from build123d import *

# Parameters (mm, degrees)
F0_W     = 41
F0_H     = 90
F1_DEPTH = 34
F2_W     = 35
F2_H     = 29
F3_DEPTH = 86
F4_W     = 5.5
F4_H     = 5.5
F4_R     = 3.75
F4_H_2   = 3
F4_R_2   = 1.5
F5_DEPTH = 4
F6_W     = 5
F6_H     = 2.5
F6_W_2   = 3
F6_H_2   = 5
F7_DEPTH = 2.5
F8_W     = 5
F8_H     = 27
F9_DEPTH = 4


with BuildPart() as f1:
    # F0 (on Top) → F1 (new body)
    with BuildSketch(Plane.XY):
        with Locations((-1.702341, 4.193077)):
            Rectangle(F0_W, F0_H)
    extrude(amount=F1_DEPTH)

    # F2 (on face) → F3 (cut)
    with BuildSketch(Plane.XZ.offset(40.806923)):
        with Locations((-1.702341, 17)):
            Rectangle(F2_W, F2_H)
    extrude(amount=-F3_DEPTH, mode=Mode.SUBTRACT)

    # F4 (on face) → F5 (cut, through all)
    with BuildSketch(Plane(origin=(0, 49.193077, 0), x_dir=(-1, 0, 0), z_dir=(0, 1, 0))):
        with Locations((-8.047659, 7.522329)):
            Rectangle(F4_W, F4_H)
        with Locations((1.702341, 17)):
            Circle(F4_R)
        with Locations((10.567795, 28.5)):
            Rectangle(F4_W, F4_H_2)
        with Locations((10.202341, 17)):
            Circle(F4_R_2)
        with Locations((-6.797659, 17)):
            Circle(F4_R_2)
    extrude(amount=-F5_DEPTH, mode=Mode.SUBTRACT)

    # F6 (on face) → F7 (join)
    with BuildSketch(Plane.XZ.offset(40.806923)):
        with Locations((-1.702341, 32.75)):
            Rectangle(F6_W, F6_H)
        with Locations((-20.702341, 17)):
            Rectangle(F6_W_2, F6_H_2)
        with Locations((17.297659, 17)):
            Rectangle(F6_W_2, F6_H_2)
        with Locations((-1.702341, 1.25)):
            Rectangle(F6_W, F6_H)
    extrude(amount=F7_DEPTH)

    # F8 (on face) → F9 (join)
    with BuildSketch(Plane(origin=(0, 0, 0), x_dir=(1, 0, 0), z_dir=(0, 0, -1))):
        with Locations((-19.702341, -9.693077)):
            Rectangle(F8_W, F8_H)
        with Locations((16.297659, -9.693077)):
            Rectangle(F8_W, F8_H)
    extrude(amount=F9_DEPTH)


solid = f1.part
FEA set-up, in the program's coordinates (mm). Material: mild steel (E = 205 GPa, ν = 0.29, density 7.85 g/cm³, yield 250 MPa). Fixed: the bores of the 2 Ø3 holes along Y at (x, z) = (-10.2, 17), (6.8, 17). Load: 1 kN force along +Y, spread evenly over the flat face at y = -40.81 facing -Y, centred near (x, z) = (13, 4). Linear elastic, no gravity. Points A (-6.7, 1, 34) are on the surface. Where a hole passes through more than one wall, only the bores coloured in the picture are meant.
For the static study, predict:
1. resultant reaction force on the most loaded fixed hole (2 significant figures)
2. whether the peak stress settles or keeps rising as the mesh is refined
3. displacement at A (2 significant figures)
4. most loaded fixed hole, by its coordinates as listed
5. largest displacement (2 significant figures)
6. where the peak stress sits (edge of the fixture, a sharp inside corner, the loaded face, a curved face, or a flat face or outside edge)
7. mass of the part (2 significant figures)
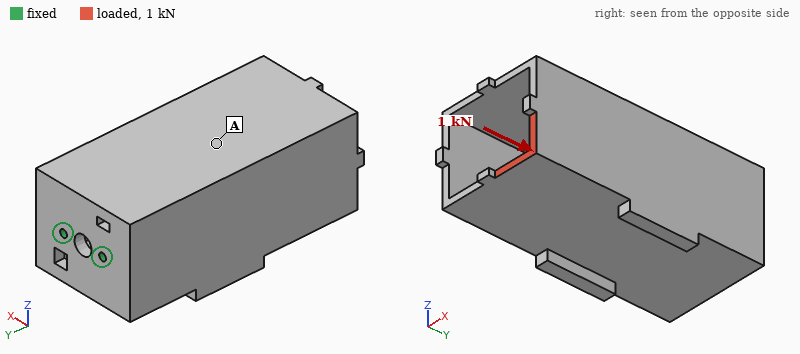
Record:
1.1 kN
keeps rising
0.061 mm
(6.8, 17)
0.12 mm
edge of the fixture
310 g
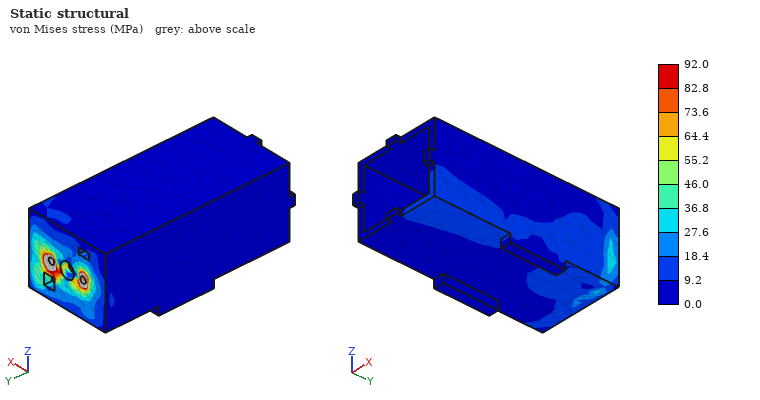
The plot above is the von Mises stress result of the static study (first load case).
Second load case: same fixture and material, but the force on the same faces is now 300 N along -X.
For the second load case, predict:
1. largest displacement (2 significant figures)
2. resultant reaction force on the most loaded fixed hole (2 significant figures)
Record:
73 µm
1.1 kN
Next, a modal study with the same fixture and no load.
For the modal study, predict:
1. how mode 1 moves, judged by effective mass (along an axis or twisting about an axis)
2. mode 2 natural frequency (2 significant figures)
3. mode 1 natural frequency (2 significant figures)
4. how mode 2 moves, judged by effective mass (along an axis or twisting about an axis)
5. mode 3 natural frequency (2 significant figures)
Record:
along Z
1100 Hz
590 Hz
along X
3200 Hz
